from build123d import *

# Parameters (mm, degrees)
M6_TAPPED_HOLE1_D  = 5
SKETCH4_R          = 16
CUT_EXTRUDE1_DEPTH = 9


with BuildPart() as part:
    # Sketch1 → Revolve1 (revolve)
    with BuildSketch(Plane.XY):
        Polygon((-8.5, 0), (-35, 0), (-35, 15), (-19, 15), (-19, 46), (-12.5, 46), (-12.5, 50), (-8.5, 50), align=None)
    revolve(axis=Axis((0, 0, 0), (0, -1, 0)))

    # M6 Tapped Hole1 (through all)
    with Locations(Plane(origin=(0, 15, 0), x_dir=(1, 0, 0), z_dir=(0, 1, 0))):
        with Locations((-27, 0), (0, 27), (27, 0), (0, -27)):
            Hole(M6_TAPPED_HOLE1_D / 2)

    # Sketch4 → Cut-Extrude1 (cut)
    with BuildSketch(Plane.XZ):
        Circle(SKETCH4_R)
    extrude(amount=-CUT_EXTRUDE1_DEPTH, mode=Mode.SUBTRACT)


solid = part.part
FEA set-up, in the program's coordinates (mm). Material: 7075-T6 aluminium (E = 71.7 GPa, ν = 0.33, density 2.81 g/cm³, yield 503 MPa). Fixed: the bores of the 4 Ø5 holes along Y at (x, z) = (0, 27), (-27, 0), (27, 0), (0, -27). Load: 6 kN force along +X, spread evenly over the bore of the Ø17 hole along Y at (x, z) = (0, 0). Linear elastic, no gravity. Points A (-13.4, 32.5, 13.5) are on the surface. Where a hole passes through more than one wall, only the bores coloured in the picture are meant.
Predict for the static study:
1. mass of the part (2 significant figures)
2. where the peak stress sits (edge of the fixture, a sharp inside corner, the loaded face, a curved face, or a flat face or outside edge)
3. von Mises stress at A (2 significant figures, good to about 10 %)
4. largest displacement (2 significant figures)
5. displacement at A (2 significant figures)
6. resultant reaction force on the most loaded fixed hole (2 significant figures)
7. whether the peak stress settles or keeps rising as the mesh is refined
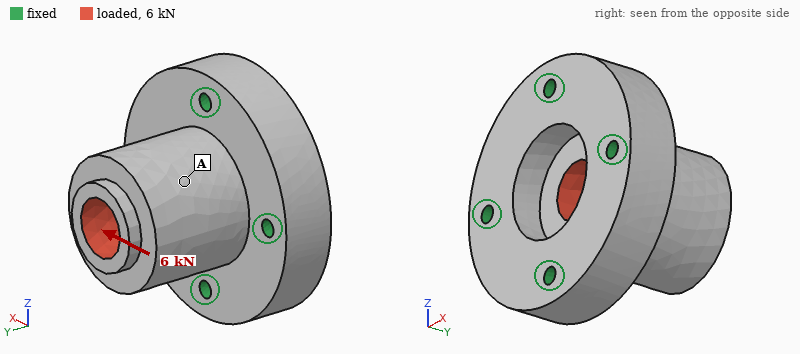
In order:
220 g
edge of the fixture
5.4 MPa
21 µm
12 µm
3.1 kN
keeps rising
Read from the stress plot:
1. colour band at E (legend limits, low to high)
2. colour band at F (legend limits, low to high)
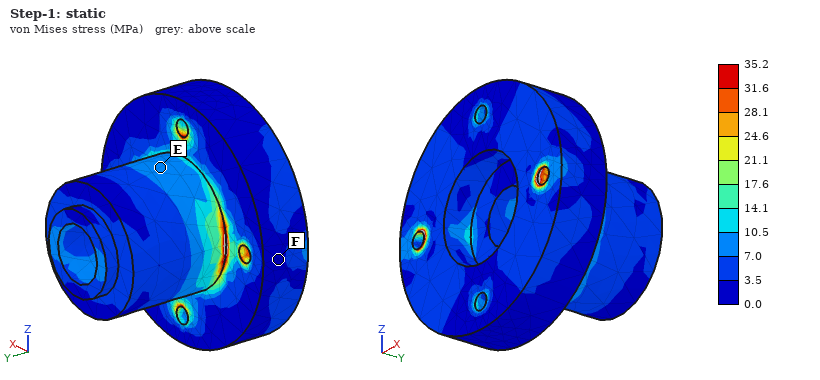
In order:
7.0 to 10.5 MPa
0.0 to 3.5 MPa
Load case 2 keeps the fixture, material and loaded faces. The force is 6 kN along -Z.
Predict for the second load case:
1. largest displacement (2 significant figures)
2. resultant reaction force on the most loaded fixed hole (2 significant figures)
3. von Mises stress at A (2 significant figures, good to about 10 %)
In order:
21 µm
3.1 kN
5.4 MPa
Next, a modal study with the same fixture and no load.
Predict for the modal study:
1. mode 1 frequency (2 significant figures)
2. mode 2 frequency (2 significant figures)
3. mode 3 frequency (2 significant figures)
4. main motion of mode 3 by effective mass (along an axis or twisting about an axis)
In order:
11 kHz
11 kHz
18 kHz
along Y
